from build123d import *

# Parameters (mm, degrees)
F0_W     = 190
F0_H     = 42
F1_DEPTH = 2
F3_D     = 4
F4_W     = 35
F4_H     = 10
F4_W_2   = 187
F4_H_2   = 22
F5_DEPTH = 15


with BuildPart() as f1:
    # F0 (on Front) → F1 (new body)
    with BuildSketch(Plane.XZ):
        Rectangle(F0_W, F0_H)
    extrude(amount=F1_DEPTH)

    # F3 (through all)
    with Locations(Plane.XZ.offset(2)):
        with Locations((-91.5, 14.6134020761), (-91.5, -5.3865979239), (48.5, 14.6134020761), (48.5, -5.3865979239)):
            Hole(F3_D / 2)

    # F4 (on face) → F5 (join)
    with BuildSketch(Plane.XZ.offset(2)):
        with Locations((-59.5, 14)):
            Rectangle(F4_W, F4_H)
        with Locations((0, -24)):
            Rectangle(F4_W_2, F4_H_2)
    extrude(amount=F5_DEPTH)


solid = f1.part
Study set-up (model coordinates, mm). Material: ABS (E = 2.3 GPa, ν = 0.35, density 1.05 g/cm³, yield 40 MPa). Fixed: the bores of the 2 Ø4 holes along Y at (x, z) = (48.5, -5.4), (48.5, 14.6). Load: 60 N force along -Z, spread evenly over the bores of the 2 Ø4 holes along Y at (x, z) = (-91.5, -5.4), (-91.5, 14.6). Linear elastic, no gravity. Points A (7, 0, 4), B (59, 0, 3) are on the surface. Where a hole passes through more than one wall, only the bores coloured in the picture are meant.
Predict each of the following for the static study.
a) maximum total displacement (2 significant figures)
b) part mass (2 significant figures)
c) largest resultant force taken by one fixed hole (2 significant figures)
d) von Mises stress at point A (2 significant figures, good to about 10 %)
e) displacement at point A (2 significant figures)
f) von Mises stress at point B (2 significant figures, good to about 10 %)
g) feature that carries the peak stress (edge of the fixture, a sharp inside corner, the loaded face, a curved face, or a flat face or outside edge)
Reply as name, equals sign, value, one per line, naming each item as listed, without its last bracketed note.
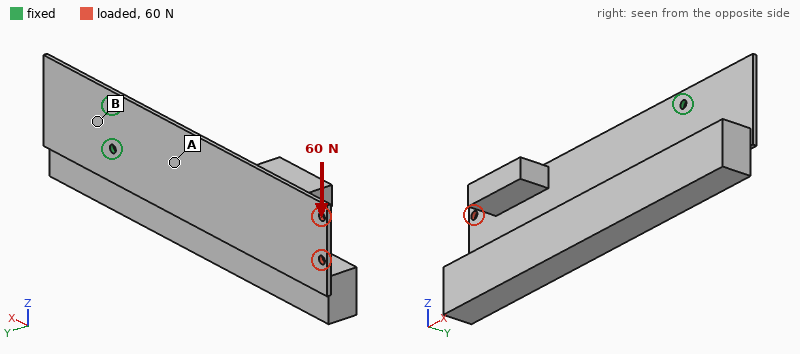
maximum total displacement = 1.6 mm
part mass = 87 g
largest resultant force taken by one fixed hole = 380 N
von Mises stress at point A = 2.1 MPa
displacement at point A = 0.31 mm
von Mises stress at point B = 4.4 MPa
feature that carries the peak stress = edge of the fixture
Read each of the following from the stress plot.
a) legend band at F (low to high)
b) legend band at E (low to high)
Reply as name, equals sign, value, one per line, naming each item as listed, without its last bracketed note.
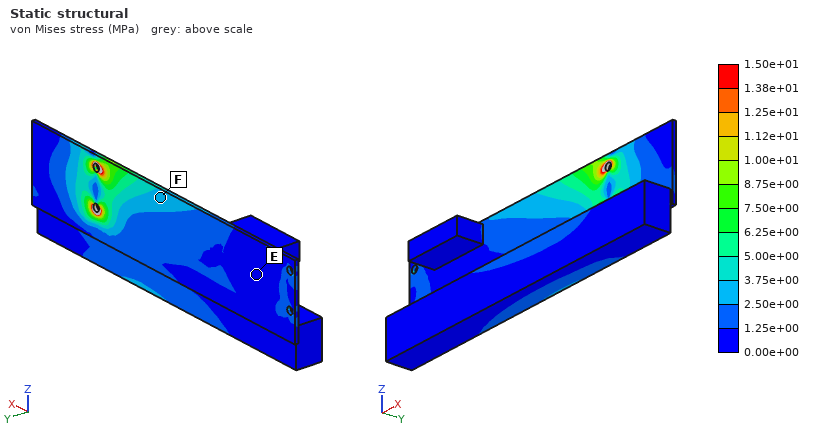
legend band at F = 2.50e+00 to 3.75e+00 MPa
legend band at E = 0.00e+00 to 1.25e+00 MPa
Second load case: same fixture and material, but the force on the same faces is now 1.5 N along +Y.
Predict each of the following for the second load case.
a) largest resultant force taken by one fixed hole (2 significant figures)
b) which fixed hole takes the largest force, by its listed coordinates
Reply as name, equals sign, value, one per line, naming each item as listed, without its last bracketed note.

largest resultant force taken by one fixed hole = 0.97 N
which fixed hole takes the largest force, by its listed coordinates = (48.5, -5.4)
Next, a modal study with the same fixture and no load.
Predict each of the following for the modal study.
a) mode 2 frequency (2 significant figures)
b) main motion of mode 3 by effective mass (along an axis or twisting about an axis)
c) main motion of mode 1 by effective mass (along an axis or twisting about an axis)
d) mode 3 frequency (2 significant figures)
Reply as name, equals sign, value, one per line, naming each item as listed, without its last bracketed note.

mode 2 frequency = 96 Hz
main motion of mode 3 by effective mass = along Z
main motion of mode 1 by effective mass = along Y
mode 3 frequency = 230 Hz
